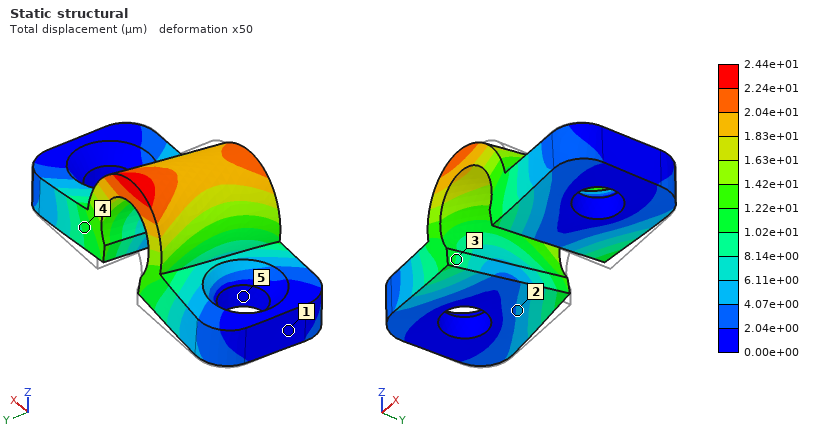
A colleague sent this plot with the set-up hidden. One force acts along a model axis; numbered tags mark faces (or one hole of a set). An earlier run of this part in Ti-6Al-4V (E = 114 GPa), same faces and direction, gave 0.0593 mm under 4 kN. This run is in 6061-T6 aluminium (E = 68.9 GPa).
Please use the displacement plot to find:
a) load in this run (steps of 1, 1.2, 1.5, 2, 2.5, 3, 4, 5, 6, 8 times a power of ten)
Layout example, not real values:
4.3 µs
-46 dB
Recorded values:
1 kN
